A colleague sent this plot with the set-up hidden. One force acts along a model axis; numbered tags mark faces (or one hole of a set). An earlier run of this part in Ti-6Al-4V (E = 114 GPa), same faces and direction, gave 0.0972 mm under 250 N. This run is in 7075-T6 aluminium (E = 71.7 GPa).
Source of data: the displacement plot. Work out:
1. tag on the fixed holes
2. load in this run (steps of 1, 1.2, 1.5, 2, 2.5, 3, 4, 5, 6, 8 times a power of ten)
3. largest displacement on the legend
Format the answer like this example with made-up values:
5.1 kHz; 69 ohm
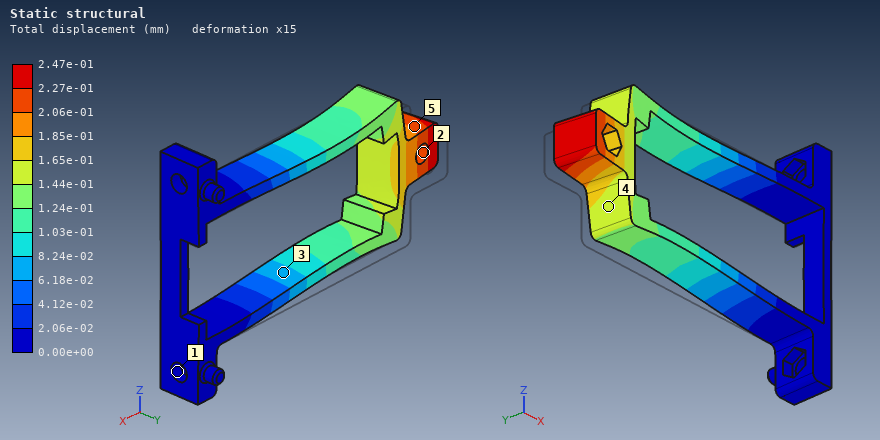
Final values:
1; 400 N; 2.47e-01 mm
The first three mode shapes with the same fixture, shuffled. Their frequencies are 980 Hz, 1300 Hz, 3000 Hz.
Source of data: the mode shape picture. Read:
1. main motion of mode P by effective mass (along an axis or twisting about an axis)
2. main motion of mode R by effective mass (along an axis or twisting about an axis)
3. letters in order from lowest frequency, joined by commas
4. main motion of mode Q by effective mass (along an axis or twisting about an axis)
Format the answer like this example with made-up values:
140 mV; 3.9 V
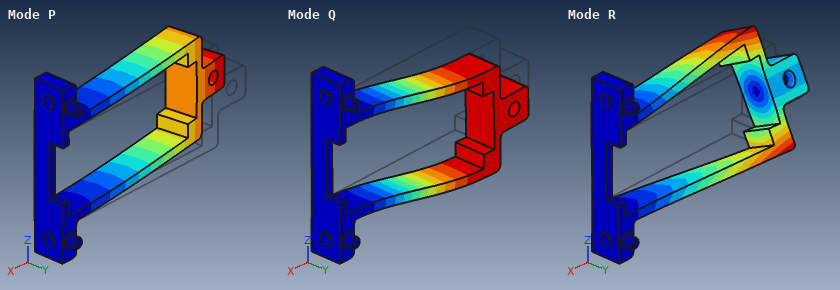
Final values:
along Y; twisting about X; Q, P, R; along Z
